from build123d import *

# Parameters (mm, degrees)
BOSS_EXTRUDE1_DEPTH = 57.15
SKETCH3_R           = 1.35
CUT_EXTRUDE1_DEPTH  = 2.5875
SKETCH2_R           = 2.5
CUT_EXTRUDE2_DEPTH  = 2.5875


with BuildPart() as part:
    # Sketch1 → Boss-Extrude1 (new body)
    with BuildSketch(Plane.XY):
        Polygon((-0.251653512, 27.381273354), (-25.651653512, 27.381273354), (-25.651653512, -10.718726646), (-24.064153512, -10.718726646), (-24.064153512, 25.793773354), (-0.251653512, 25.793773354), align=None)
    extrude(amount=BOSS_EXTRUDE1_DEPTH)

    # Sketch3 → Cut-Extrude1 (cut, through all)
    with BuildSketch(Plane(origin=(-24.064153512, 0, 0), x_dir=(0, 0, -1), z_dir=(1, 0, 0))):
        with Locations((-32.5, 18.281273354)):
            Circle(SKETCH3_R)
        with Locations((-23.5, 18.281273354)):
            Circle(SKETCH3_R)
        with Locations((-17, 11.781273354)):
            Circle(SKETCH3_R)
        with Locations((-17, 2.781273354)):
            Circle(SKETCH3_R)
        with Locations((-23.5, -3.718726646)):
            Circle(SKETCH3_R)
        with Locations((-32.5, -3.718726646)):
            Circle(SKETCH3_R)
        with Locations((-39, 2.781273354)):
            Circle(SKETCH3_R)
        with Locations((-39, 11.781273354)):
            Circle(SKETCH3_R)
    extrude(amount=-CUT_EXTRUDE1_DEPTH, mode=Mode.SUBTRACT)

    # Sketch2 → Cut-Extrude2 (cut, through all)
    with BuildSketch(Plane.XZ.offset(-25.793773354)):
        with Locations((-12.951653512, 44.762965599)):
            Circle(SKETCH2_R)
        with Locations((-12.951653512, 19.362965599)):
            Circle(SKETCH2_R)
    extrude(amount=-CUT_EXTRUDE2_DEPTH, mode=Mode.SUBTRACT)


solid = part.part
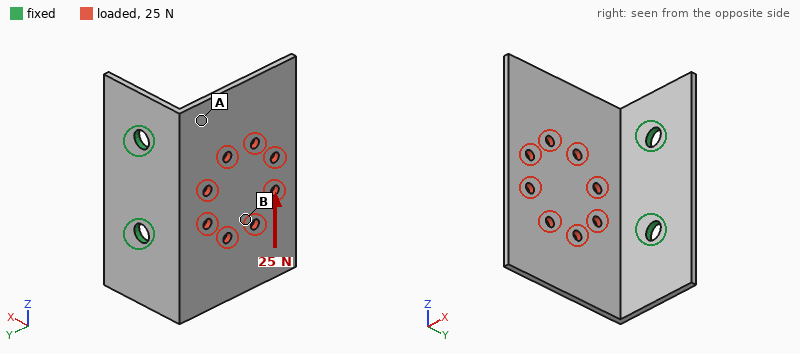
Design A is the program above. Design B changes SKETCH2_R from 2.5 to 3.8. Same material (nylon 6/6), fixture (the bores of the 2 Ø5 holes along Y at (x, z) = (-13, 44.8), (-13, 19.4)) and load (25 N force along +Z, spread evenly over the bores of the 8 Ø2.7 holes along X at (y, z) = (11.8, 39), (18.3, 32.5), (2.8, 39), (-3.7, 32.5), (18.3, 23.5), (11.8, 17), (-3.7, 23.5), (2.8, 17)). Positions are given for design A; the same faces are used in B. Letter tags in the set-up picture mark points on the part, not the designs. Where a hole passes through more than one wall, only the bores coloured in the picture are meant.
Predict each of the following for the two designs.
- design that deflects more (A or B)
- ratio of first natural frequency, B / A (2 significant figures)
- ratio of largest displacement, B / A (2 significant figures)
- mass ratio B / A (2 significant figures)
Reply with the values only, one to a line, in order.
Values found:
A
1.1
0.74
0.99
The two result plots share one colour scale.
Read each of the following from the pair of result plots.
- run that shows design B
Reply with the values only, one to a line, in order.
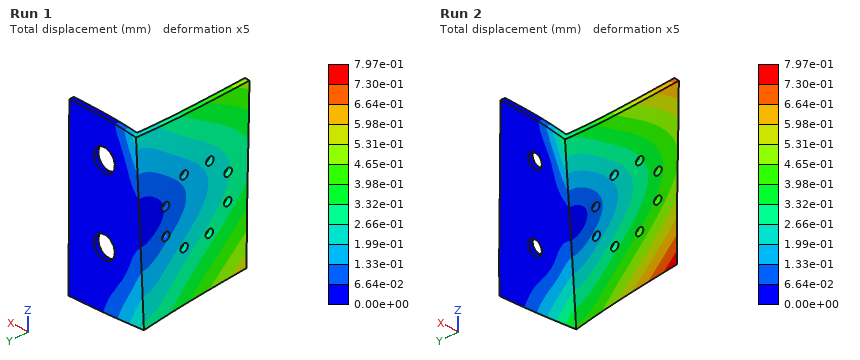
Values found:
Run 1
